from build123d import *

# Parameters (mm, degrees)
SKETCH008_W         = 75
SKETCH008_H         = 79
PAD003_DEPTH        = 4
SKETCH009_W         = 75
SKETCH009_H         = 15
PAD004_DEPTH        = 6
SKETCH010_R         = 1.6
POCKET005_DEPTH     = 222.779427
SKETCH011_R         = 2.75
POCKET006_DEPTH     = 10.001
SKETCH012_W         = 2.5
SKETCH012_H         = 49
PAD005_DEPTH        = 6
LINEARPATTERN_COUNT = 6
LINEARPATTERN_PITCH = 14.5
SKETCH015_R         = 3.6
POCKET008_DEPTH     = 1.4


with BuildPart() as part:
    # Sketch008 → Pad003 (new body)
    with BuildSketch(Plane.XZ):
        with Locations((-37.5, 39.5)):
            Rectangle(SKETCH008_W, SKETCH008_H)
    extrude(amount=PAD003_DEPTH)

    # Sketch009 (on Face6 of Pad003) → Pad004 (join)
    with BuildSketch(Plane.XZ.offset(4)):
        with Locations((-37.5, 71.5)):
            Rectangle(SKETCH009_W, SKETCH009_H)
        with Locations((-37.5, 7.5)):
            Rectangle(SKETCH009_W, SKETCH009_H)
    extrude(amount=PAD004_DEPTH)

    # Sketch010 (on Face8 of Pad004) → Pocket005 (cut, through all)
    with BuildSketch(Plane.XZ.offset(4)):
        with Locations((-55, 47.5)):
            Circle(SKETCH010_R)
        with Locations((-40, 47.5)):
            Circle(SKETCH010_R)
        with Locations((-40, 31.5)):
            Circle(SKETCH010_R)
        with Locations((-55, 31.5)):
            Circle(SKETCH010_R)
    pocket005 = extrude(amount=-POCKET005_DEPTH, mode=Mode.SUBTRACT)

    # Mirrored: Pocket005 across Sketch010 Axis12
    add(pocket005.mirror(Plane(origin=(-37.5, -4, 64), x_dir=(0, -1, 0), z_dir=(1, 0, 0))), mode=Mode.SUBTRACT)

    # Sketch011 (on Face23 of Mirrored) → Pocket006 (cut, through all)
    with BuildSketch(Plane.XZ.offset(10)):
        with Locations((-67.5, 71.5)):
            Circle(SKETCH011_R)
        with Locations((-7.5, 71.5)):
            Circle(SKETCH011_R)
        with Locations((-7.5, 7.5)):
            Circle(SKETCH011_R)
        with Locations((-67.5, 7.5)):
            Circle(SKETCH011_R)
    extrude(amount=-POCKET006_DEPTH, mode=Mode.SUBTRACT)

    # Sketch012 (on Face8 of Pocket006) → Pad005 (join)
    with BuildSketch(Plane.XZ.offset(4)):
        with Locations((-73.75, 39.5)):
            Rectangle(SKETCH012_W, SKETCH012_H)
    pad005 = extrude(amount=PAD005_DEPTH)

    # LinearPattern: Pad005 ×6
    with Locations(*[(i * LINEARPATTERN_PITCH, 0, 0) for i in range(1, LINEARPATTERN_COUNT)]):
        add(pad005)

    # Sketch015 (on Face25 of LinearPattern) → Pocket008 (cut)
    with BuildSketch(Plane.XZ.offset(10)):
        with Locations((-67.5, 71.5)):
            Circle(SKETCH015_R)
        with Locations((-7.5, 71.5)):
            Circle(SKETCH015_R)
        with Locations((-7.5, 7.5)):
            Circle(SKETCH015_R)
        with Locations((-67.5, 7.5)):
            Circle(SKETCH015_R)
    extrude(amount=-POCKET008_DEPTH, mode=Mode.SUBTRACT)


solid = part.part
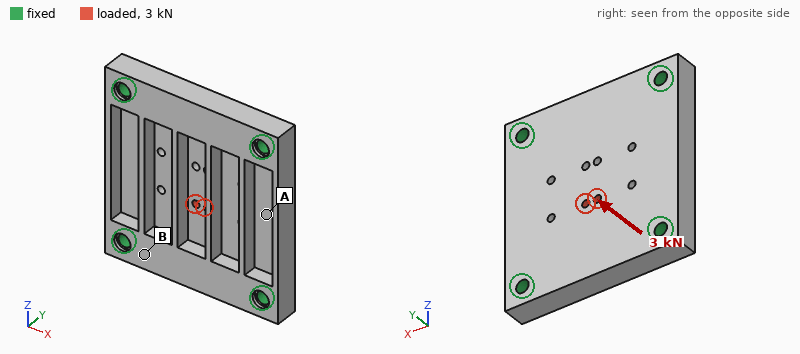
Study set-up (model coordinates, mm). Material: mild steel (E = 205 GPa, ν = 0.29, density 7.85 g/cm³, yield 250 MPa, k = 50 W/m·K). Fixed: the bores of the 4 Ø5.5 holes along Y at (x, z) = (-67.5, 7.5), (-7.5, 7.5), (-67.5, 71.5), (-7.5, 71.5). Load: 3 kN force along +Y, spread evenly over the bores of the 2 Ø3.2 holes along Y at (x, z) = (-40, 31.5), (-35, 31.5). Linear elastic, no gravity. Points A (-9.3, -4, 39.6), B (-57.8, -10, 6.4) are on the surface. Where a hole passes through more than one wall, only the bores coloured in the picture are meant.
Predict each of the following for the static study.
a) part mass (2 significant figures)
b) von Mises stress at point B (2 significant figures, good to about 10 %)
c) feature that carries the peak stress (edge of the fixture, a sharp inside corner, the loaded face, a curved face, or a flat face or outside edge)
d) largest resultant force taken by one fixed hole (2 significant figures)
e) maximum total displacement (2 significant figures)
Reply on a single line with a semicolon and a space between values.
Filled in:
320 g; 43 MPa; the loaded face; 1.1 kN; 44 µm
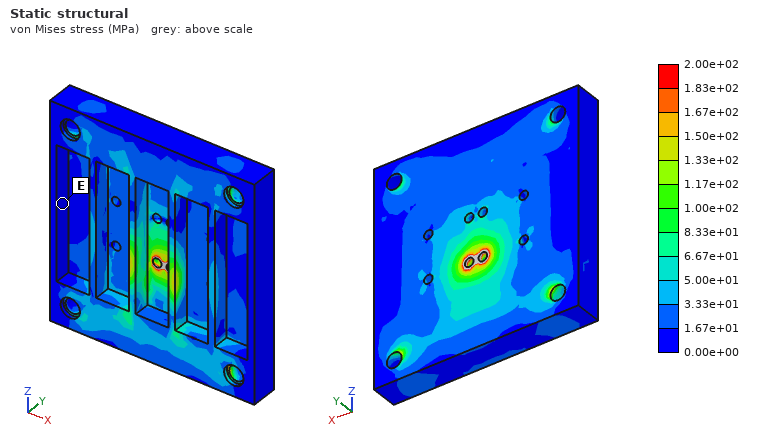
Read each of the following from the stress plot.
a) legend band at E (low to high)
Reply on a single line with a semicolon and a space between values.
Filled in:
0.00e+00 to 1.67e+01 MPa
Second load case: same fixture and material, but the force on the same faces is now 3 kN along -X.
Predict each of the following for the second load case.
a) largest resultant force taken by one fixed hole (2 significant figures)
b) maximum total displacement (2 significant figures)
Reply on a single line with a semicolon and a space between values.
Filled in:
1.1 kN; 4.4 µm
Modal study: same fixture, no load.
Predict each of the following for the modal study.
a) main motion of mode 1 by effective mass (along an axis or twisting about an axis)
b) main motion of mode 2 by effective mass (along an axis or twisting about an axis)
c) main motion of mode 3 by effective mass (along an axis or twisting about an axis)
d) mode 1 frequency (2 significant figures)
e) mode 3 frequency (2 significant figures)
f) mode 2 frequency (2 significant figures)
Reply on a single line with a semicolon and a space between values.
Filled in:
along Y; twisting about Z; twisting about X; 7200 Hz; 12 kHz; 11 kHz
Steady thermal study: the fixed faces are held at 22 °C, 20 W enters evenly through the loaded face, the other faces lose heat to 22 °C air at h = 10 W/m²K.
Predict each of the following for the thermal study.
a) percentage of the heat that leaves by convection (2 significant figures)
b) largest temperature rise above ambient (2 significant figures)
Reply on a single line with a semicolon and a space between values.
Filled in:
7.6 %; 50 K
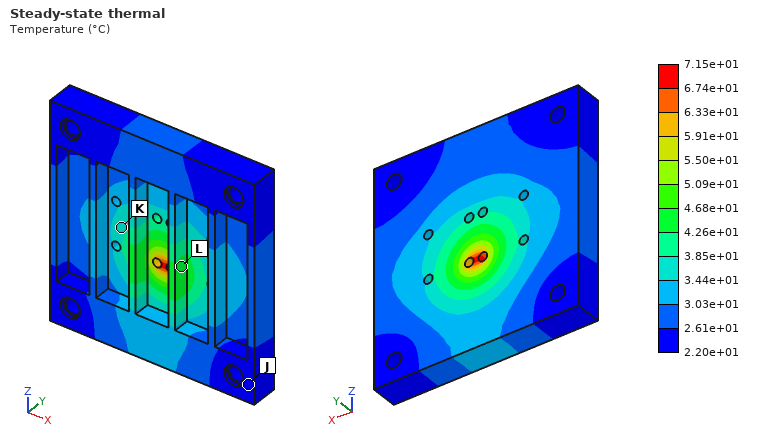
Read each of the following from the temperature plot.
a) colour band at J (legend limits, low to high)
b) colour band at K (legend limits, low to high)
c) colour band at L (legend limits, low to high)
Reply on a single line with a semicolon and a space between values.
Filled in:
2.20e+01 to 2.61e+01 °C; 3.44e+01 to 3.85e+01 °C; 4.26e+01 to 4.68e+01 °C
